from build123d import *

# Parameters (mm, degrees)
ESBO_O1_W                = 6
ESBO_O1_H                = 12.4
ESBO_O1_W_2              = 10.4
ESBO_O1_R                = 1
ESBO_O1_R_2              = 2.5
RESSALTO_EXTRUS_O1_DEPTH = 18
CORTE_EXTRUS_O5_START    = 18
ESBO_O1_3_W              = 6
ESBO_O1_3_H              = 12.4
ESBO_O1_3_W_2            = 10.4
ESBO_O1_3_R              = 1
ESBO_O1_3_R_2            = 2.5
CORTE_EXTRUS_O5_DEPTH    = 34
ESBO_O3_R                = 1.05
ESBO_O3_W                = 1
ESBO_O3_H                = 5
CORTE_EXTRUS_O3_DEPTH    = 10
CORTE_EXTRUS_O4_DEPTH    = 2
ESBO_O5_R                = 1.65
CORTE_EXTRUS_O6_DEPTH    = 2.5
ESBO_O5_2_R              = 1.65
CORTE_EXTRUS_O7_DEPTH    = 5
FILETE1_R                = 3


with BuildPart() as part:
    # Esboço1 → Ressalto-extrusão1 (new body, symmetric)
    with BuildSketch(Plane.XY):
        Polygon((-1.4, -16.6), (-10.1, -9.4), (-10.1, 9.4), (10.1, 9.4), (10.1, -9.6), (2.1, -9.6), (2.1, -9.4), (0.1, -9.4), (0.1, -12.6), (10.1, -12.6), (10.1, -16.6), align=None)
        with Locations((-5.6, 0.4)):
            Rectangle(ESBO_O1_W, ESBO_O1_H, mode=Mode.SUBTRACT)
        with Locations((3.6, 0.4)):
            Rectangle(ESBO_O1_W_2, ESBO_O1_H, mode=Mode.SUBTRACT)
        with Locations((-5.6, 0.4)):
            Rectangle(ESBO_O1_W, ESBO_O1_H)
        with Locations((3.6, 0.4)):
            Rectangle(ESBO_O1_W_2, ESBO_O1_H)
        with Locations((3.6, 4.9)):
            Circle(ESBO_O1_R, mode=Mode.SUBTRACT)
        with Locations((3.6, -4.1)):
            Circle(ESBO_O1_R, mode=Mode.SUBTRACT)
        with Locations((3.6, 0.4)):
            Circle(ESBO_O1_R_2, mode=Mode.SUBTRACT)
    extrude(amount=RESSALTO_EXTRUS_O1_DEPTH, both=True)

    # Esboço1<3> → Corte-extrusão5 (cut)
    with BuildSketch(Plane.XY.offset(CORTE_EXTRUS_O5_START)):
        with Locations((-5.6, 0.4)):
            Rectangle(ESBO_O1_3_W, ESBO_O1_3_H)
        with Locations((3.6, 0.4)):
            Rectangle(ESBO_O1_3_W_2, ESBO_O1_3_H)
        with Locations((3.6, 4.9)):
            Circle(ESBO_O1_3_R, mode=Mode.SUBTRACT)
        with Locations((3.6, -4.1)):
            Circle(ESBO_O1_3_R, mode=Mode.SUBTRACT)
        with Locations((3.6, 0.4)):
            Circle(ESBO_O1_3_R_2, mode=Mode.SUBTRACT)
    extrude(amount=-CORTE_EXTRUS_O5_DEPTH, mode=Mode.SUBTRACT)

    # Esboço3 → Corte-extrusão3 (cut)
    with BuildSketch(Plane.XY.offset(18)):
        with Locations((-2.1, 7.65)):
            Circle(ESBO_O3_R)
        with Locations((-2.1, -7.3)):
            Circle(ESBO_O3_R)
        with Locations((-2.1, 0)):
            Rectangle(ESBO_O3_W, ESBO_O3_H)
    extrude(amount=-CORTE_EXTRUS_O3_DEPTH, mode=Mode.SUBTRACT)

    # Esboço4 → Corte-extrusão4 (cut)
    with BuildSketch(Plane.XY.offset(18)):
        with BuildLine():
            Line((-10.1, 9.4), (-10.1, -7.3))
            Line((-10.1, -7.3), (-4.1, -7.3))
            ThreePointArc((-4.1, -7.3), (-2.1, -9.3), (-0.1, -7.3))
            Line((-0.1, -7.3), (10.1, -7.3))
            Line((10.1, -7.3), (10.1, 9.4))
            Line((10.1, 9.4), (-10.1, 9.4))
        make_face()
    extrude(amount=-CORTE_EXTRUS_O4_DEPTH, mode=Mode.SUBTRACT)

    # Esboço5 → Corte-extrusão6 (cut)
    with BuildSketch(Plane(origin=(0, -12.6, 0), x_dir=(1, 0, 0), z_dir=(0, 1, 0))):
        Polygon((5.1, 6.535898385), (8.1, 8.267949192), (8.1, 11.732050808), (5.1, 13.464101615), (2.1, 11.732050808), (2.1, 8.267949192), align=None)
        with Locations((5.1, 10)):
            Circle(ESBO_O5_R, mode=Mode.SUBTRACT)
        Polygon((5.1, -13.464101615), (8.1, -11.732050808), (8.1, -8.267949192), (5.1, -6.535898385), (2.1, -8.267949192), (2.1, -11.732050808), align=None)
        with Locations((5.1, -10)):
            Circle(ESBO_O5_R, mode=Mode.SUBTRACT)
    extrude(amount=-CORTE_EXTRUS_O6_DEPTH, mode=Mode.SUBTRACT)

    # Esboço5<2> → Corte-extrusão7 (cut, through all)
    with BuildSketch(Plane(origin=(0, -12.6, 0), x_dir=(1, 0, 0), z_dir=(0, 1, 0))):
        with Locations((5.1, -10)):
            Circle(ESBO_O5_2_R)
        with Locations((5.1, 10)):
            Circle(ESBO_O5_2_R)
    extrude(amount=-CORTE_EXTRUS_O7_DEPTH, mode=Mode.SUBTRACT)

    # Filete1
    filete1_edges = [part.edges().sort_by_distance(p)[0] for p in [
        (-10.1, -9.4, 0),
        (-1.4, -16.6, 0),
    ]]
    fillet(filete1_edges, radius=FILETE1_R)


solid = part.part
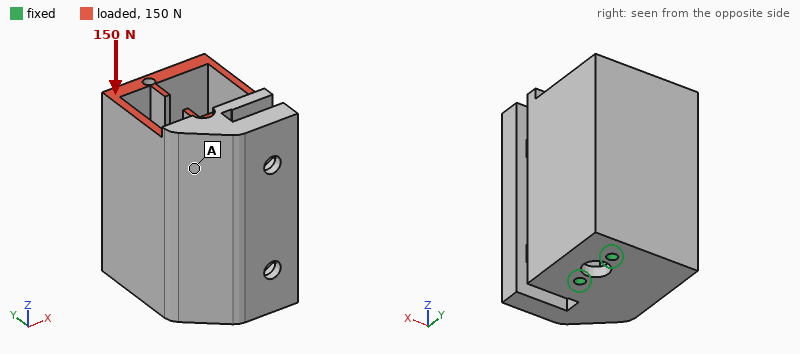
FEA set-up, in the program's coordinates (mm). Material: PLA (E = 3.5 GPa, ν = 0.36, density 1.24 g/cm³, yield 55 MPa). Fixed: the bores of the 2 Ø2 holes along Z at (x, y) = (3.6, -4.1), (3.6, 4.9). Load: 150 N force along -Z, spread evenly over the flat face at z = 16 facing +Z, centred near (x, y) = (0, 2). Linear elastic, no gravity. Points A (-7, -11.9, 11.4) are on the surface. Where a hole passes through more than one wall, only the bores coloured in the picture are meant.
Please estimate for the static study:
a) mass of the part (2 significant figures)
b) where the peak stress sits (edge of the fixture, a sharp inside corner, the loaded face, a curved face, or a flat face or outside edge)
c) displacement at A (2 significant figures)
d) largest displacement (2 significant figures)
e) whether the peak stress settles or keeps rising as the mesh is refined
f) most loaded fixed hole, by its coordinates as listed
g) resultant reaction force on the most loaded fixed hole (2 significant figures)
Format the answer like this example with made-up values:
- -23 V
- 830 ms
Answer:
- 11 g
- edge of the fixture
- 0.45 mm
- 0.56 mm
- keeps rising
- (3.6, 4.9)
- 92 N
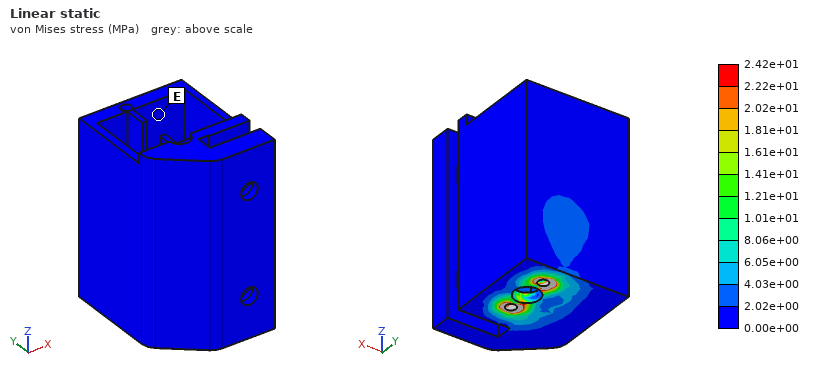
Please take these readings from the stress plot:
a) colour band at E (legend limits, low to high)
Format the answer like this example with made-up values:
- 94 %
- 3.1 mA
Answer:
- 0.00e+00 to 2.02e+00 MPa
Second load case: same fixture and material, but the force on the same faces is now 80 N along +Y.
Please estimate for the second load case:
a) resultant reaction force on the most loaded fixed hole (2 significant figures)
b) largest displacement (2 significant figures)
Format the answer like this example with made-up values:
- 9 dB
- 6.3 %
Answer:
- 220 N
- 0.51 mm
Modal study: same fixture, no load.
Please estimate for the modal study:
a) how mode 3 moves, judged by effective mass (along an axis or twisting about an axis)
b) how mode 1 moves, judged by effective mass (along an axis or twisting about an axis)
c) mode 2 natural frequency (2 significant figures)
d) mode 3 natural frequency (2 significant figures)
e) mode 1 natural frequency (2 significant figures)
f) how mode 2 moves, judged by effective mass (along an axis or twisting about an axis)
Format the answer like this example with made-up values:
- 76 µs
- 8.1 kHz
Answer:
- twisting about Z
- along X
- 1000 Hz
- 2600 Hz
- 460 Hz
- along Y
